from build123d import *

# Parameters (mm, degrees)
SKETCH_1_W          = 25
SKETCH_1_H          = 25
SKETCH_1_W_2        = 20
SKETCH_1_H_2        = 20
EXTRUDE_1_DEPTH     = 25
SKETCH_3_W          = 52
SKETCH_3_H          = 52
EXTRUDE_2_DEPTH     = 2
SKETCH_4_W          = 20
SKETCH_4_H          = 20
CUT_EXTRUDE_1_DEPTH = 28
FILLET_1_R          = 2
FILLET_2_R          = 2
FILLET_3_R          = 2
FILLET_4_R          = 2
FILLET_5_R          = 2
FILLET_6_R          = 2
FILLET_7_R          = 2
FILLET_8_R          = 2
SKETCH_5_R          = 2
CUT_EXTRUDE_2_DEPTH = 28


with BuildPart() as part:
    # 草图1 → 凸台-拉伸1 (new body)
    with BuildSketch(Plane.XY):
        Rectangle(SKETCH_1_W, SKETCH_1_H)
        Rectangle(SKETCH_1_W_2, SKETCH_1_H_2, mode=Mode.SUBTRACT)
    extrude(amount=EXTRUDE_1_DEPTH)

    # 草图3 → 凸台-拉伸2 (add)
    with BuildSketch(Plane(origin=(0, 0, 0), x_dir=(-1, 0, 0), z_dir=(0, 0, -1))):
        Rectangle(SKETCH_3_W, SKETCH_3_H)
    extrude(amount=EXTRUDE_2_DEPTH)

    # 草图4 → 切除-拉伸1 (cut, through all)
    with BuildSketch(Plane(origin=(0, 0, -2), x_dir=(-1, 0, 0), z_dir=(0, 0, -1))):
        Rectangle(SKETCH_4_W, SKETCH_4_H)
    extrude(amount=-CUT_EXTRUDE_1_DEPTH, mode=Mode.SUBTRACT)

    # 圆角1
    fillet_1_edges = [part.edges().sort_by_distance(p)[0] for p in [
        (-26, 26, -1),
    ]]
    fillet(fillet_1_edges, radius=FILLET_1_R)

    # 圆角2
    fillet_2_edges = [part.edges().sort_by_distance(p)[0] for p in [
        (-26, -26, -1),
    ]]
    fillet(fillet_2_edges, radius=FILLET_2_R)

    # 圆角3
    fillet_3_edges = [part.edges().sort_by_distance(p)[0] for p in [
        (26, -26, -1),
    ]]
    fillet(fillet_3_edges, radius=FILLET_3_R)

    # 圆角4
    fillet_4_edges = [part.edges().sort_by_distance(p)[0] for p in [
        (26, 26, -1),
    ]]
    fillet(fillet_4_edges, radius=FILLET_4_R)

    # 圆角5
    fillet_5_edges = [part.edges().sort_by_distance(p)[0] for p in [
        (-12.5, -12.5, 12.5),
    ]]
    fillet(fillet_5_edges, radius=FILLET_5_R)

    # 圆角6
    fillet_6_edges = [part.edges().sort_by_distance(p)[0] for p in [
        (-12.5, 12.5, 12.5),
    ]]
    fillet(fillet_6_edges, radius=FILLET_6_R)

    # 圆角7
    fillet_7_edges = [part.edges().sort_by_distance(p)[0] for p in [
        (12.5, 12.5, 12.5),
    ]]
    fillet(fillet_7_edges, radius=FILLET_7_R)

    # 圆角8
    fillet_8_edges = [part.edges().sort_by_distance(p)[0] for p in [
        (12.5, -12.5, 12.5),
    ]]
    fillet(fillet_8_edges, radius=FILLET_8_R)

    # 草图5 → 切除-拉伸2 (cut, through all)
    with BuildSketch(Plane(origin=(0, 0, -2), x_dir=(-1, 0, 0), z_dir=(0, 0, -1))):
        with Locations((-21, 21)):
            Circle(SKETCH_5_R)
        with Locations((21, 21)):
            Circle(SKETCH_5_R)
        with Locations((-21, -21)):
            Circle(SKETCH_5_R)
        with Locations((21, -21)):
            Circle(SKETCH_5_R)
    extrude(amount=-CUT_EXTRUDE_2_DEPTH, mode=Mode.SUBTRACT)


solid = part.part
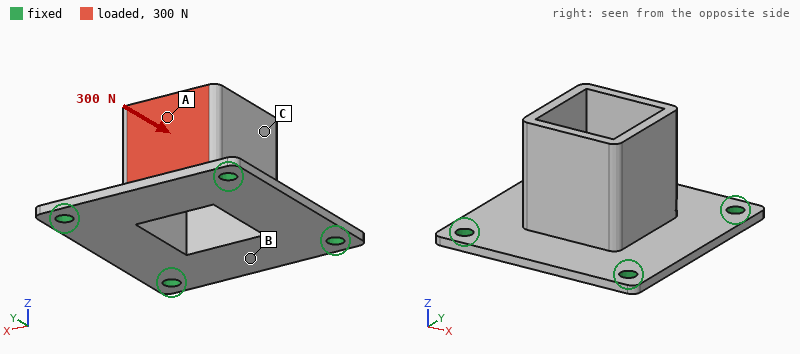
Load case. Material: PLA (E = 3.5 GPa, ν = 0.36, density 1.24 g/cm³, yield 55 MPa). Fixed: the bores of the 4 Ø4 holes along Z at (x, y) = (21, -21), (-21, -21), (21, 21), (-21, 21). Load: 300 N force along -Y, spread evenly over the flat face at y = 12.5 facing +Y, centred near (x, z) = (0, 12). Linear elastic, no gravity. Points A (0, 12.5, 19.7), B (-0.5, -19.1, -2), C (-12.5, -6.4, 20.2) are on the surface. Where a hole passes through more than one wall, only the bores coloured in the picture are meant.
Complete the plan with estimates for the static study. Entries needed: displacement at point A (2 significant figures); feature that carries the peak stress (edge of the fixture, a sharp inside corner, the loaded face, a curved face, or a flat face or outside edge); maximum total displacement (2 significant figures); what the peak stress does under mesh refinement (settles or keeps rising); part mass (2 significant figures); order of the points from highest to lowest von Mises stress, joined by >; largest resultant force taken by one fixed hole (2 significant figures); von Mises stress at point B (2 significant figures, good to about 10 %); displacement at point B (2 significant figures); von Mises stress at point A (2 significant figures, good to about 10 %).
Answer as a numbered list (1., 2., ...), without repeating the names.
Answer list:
1. 0.73 mm
2. edge of the fixture
3. 0.89 mm
4. keeps rising
5. 12 g
6. A > B > C
7. 110 N
8. 7.6 MPa
9. 0.31 mm
10. 16 MPa
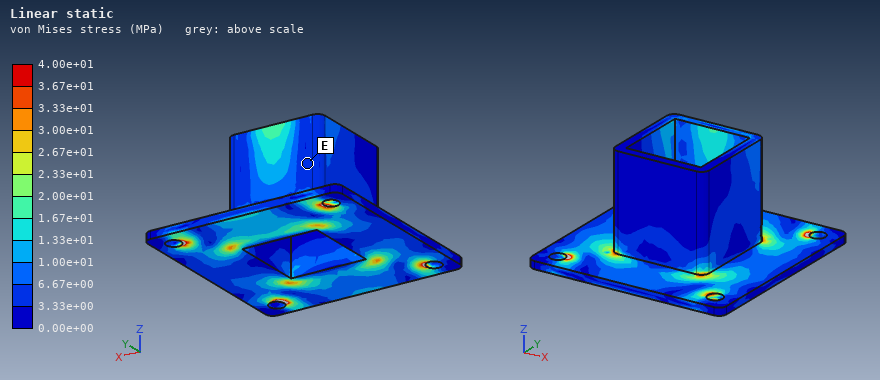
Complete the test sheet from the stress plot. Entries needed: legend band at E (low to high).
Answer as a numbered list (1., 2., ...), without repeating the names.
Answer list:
1. 3.33e+00 to 6.67e+00 MPa
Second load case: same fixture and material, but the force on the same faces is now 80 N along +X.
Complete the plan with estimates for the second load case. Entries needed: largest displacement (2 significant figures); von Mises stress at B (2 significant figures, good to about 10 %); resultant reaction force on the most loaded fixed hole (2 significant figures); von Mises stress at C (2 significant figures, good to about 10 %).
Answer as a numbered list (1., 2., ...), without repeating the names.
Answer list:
1. 0.22 mm
2. 1.6 MPa
3. 37 N
4. 1.3 MPa
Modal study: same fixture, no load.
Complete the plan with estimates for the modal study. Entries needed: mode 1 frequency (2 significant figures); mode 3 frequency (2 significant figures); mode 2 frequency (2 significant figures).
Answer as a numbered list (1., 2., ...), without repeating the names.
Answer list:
1. 1300 Hz
2. 1300 Hz
3. 1300 Hz
